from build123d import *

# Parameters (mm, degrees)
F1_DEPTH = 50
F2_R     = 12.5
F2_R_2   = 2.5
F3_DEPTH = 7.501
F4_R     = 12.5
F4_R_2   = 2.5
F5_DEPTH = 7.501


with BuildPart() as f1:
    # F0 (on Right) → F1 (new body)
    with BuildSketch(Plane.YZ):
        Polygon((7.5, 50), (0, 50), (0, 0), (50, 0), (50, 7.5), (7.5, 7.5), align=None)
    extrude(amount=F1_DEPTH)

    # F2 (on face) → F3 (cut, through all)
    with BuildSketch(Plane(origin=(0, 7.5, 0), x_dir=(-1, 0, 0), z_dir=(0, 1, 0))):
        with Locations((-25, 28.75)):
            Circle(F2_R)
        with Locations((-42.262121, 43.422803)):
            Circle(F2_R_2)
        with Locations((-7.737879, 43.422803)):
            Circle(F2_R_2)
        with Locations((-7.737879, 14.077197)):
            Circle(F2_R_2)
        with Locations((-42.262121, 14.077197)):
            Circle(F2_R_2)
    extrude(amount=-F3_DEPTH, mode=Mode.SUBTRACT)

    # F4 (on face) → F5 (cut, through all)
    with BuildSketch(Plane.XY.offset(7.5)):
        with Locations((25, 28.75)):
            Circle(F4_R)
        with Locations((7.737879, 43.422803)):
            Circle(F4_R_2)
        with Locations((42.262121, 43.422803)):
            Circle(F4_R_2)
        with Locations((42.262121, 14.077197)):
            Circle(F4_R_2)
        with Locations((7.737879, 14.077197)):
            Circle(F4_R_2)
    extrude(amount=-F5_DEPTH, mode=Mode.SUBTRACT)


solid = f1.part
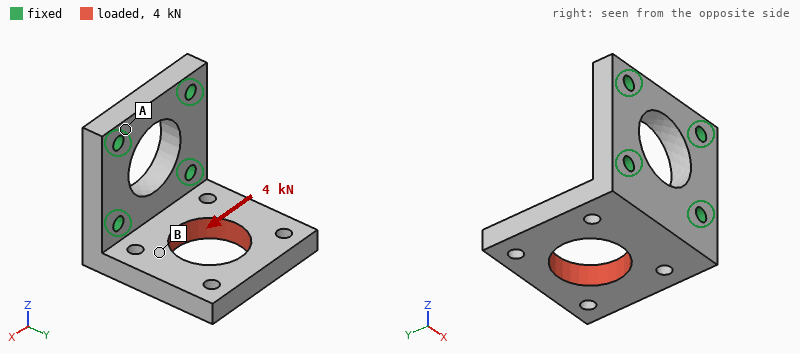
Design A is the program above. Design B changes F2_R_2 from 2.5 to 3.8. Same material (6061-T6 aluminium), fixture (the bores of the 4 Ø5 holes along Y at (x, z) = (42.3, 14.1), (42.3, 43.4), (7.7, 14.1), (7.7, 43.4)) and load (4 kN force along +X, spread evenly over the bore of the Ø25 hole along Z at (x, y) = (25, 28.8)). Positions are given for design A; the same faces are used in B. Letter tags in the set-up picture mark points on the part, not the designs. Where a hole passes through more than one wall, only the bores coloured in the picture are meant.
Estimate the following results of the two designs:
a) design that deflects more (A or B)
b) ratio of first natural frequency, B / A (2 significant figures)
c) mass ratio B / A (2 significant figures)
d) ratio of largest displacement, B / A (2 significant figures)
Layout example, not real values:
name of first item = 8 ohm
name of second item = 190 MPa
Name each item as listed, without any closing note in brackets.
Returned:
design that deflects more = A
ratio of first natural frequency, B / A = 1.0
mass ratio B / A = 0.97
ratio of largest displacement, B / A = 0.84
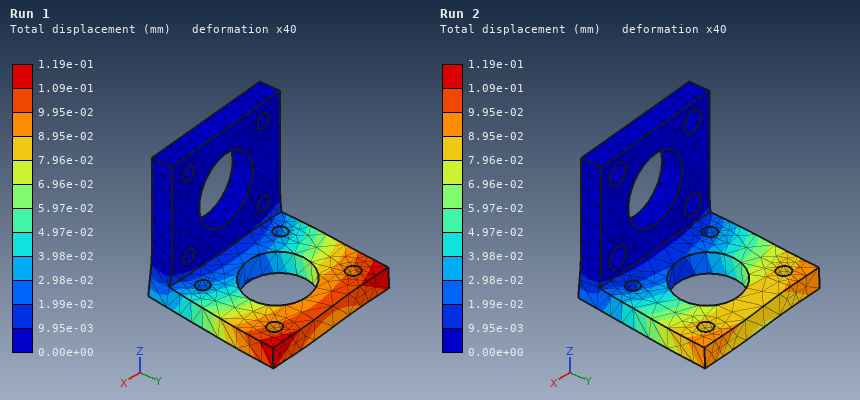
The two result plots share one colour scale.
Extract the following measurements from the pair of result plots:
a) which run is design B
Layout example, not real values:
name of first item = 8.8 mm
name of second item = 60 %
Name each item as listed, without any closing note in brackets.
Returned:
which run is design B = Run 2
